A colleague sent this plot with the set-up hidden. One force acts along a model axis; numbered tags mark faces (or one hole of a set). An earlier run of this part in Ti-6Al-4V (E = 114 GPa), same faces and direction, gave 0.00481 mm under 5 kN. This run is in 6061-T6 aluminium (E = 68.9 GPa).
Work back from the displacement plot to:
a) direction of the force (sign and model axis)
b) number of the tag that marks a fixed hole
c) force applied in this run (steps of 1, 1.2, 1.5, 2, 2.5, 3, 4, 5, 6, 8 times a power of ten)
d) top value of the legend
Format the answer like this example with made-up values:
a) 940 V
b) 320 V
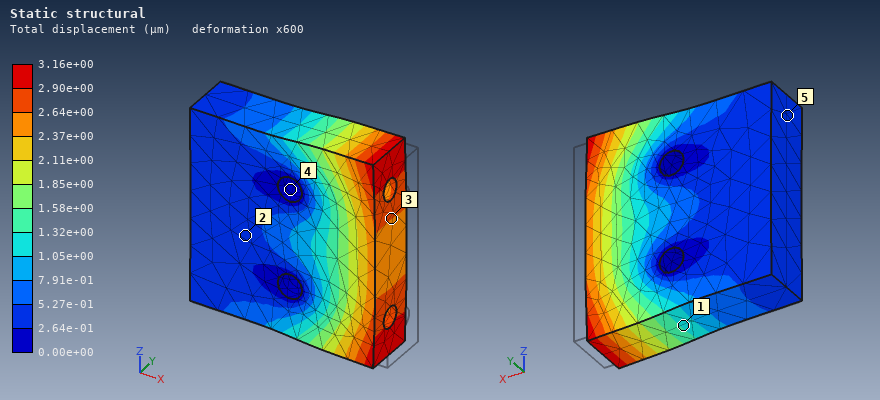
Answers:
a) -X
b) 4
c) 2 kN
d) 3.16e+00 µm
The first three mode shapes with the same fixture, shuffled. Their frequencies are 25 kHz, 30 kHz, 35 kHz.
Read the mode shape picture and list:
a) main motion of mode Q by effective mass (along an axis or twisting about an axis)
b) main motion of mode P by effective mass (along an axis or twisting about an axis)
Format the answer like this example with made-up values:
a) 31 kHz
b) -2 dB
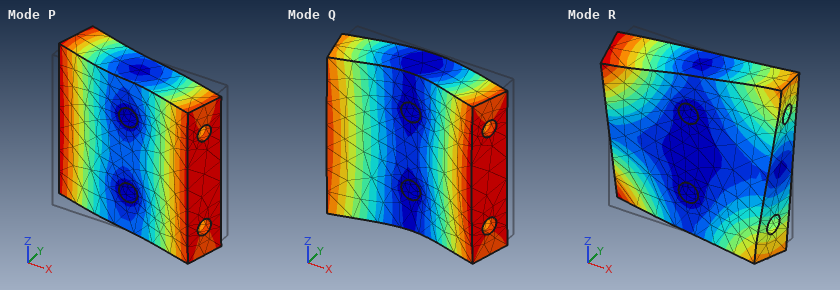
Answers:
a) along Y
b) twisting about Z
